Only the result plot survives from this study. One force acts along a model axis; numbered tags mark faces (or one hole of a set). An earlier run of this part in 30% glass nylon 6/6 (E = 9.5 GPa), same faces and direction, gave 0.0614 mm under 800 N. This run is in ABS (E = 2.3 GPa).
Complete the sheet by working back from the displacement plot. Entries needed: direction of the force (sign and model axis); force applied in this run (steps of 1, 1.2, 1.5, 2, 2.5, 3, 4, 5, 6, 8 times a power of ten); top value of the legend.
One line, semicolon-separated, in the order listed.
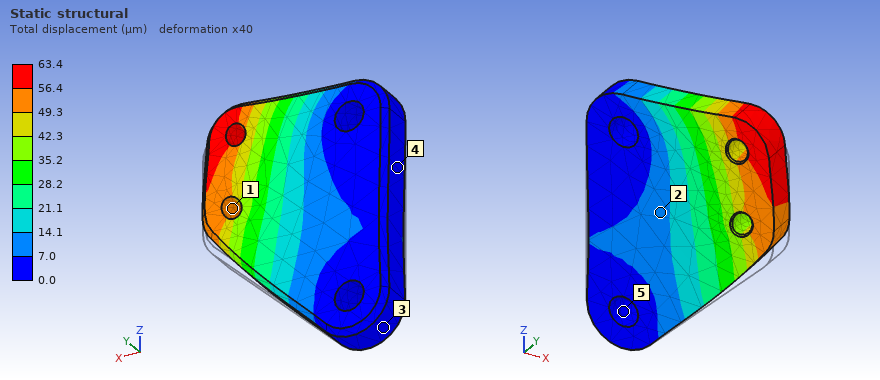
+Z; 200 N; 63.4 µm
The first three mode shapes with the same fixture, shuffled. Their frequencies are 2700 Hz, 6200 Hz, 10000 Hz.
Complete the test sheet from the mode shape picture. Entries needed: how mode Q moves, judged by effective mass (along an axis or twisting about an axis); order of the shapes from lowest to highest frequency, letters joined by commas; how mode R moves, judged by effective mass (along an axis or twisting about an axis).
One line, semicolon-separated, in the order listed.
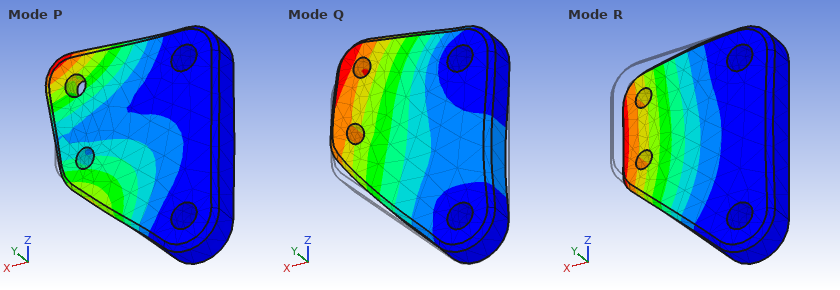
along Z; R, P, Q; along Y
